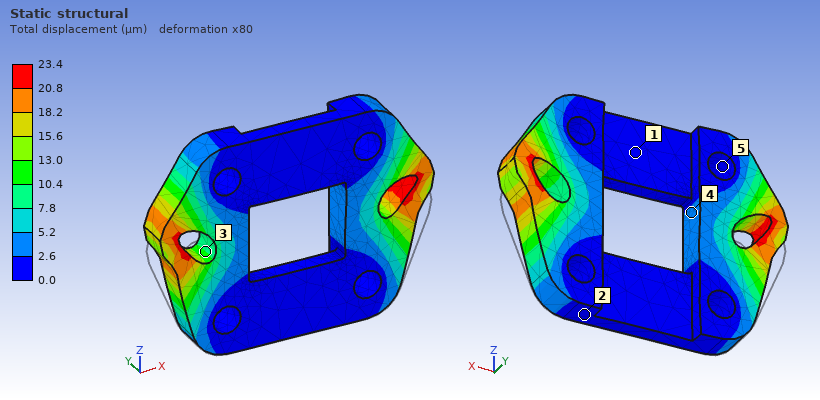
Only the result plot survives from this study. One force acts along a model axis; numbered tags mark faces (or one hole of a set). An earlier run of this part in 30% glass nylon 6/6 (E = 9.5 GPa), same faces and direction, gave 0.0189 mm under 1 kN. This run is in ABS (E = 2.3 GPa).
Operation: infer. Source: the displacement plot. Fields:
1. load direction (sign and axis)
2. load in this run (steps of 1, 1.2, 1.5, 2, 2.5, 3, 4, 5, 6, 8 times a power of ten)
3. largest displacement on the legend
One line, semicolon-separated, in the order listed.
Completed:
+Z; 300 N; 23.4 µm
